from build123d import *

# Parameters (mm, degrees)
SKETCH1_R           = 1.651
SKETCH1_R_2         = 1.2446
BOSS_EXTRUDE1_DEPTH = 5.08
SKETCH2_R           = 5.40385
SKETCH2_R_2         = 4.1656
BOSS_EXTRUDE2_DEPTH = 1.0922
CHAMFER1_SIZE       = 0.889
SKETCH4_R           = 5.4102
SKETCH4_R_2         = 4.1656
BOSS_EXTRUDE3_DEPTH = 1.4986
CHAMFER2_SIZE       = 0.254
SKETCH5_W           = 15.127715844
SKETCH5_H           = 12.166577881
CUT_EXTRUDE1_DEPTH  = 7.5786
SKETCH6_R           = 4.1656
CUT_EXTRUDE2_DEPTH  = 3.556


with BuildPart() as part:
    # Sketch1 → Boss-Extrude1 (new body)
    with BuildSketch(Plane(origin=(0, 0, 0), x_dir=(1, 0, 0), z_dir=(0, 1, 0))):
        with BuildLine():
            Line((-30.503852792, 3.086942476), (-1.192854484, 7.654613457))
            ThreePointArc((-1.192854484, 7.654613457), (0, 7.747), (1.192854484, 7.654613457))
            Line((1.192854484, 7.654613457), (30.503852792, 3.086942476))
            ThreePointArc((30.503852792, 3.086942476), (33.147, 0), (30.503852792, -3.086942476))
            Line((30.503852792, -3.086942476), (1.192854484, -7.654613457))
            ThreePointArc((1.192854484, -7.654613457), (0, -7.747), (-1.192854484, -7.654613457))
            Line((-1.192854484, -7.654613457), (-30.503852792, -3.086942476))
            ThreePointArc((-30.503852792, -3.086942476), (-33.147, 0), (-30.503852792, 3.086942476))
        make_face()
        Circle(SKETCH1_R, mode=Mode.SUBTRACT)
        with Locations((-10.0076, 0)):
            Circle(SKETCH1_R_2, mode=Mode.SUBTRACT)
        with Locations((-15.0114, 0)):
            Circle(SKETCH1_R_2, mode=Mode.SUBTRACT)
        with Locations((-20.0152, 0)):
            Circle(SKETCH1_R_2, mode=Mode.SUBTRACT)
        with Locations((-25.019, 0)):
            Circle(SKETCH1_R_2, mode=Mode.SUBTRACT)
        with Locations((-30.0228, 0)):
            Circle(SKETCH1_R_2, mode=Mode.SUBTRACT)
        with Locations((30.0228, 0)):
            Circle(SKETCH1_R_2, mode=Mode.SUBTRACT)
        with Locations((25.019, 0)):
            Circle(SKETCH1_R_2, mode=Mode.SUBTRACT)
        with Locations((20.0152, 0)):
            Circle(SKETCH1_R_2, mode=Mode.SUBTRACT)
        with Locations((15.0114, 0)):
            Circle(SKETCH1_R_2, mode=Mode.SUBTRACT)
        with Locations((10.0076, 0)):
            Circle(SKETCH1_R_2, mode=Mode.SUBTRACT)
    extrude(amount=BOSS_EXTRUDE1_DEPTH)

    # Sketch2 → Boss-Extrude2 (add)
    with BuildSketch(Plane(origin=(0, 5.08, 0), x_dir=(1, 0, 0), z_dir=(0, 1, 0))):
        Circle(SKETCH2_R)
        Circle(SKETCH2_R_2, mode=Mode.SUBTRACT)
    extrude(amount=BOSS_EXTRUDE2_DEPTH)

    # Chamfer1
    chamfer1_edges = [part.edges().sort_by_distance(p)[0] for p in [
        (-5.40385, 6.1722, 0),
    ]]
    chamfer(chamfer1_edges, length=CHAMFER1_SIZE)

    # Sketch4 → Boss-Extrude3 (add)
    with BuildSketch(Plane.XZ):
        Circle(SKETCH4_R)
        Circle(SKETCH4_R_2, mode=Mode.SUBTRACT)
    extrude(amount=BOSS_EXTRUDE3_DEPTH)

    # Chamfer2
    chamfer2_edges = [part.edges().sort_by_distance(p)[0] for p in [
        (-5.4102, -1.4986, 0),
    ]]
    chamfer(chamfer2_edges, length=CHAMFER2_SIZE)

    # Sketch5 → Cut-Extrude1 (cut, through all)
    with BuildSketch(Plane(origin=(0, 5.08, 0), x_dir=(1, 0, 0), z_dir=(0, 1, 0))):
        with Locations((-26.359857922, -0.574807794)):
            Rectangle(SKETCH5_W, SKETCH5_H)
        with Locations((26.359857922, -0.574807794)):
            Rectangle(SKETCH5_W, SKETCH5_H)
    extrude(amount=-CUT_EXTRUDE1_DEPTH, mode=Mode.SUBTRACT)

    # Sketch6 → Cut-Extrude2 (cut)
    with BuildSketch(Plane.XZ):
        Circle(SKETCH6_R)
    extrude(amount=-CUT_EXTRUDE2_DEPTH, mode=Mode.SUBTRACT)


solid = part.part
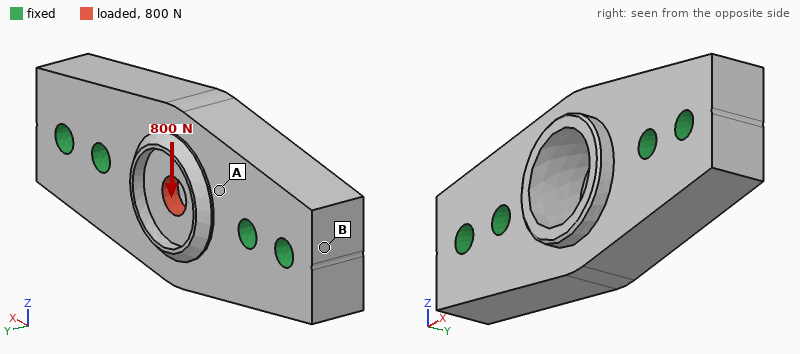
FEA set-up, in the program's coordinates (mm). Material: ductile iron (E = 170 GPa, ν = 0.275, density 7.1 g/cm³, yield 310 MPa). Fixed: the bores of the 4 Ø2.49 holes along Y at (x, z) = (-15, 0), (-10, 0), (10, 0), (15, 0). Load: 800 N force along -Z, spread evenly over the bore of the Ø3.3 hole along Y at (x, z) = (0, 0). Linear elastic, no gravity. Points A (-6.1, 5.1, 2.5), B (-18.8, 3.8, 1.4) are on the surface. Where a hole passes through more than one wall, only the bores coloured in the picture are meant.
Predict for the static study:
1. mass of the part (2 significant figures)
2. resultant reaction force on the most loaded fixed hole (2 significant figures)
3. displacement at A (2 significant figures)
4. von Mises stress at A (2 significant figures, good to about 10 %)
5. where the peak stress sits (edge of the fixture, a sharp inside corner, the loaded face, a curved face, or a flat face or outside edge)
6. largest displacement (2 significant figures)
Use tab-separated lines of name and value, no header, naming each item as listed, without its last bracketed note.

mass of the part	16 g
resultant reaction force on the most loaded fixed hole	480 N
displacement at A	0.86 µm
von Mises stress at A	22 MPa
where the peak stress sits	the loaded face
largest displacement	2.4 µm
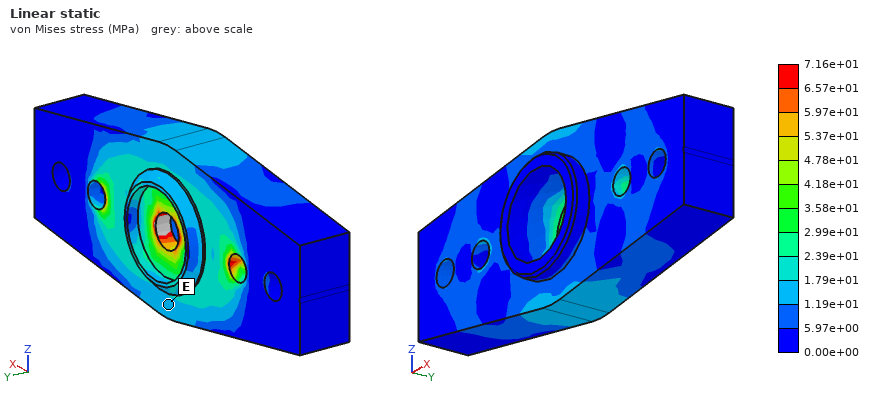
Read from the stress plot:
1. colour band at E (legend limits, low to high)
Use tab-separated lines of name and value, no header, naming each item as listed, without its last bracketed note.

colour band at E	1.19e+01 to 1.79e+01 MPa
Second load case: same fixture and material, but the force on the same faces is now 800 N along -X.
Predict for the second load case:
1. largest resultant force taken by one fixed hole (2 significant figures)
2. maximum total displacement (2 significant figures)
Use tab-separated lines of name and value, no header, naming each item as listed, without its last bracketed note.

largest resultant force taken by one fixed hole	310 N
maximum total displacement	1.4 µm
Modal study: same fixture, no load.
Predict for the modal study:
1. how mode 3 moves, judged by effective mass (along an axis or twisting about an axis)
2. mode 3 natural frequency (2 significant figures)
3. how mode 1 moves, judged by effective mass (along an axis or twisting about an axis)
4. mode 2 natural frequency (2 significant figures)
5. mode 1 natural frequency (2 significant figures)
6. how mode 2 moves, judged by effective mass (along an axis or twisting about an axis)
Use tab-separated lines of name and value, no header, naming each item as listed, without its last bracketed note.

how mode 3 moves, judged by effective mass	along Z
mode 3 natural frequency	62 kHz
how mode 1 moves, judged by effective mass	twisting about X
mode 2 natural frequency	41 kHz
mode 1 natural frequency	39 kHz
how mode 2 moves, judged by effective mass	along Y
